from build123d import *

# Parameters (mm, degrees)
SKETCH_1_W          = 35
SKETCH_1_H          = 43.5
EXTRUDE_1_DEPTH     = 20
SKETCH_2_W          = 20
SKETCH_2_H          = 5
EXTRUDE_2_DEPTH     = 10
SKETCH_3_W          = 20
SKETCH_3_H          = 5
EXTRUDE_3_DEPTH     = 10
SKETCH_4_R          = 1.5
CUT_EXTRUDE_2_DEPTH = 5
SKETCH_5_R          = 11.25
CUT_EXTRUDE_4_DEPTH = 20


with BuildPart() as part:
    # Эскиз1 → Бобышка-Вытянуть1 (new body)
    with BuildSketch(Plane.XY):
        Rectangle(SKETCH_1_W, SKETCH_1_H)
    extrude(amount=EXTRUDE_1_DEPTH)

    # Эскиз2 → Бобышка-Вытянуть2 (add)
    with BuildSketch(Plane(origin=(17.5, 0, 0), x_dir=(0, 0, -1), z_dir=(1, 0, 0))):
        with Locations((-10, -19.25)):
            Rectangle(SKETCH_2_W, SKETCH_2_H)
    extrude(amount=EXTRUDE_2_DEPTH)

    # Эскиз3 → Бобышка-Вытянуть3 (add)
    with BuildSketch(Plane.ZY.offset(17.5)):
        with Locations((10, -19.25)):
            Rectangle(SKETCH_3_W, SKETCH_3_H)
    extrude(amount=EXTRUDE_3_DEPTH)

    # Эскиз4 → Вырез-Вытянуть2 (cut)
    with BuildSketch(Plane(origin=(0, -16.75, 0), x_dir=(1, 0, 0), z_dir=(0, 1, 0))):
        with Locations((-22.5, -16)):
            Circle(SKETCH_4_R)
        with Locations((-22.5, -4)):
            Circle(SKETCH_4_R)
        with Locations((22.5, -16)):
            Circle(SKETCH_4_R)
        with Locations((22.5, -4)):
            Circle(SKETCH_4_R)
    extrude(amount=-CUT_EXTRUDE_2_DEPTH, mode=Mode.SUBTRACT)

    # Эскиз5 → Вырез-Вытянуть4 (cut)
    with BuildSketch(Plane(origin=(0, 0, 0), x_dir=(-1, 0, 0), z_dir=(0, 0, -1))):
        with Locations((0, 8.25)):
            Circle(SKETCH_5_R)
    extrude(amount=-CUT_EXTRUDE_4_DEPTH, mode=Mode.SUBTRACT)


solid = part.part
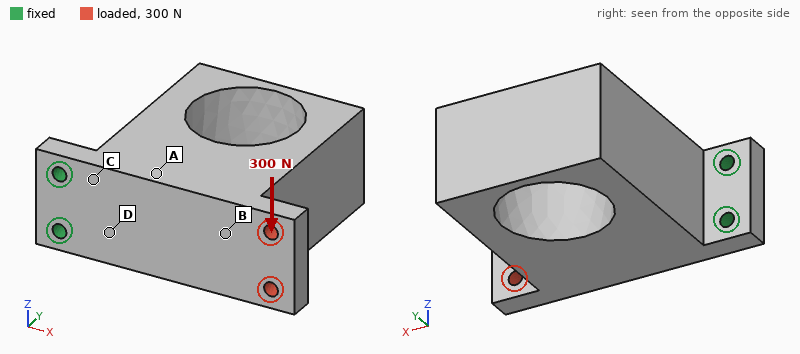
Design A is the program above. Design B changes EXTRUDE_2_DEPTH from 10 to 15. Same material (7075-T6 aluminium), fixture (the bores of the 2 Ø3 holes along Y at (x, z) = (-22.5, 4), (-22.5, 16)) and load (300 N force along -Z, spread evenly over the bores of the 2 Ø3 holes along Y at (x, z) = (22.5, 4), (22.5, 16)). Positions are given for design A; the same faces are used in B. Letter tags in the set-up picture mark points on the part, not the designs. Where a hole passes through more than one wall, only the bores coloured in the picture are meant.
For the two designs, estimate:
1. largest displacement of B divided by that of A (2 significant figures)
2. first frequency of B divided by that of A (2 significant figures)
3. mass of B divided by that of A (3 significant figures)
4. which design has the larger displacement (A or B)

1.1
0.98
1.02
B
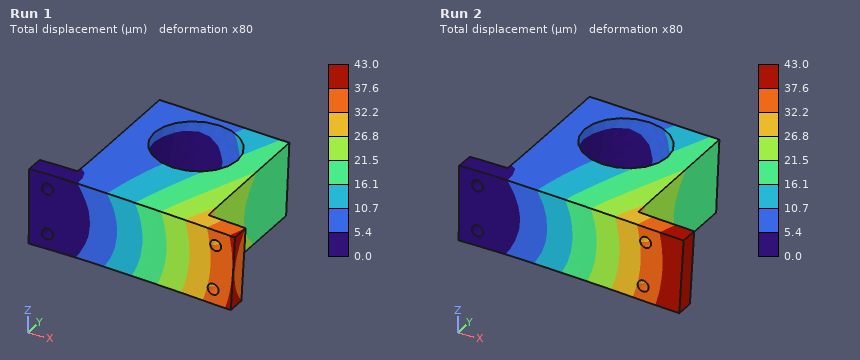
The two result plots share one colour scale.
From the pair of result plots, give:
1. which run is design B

Run 2
